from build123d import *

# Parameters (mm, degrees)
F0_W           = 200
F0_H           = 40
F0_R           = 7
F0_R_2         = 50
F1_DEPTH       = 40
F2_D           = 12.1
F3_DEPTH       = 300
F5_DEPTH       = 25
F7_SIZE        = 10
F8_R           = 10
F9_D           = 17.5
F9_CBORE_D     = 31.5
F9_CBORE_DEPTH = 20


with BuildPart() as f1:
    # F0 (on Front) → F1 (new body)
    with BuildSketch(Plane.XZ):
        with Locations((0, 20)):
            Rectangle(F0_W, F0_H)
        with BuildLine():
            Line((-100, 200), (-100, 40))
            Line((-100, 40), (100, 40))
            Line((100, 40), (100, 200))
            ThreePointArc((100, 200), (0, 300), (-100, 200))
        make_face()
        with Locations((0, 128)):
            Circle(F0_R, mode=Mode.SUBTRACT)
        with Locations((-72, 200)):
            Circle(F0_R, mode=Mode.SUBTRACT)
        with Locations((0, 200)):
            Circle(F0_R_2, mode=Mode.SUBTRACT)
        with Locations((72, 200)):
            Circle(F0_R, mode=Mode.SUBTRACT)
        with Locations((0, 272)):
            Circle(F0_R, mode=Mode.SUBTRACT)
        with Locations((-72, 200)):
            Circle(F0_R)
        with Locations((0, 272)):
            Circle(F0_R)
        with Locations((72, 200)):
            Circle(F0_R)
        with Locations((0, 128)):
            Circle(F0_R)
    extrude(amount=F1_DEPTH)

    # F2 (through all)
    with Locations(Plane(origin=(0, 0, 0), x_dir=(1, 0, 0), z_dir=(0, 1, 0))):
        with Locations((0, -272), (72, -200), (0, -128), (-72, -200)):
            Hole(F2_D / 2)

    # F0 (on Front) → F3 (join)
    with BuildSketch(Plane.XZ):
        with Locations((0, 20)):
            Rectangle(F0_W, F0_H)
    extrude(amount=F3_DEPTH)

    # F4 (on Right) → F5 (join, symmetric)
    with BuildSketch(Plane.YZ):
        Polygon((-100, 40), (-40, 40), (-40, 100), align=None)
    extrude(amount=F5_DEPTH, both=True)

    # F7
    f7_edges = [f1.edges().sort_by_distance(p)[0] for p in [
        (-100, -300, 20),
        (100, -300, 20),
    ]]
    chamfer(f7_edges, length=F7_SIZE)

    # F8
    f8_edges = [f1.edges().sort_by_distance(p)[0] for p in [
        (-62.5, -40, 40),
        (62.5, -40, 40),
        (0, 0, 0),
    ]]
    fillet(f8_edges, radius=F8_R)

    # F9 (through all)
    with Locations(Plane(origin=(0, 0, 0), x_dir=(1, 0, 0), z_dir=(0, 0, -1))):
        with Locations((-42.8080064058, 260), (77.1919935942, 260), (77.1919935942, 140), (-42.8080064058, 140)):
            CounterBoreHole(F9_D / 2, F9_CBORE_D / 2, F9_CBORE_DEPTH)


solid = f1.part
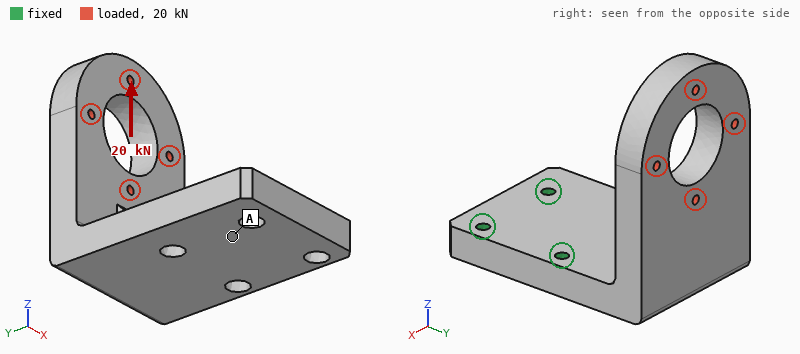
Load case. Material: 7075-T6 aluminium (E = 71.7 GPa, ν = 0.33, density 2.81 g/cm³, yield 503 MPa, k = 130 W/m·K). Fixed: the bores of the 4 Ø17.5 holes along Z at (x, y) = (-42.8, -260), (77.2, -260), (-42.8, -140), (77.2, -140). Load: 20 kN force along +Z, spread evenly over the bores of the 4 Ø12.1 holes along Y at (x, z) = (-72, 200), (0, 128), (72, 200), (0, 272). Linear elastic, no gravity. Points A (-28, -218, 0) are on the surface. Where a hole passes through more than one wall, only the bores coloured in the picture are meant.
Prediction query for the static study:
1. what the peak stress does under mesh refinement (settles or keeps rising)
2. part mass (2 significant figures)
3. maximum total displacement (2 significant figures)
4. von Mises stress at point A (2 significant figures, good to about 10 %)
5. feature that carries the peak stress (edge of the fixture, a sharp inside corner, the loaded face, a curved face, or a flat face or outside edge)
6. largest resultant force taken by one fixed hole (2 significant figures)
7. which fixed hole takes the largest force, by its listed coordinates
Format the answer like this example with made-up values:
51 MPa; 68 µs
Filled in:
keeps rising; 11 kg; 0.77 mm; 8.3 MPa; edge of the fixture; 25 kN; (-42.8, -140)
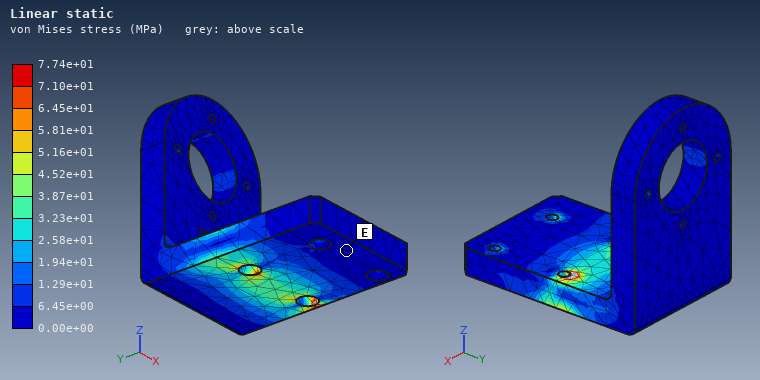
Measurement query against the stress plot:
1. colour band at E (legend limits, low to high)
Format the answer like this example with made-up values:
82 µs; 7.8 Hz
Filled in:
0.00e+00 to 6.45e+00 MPa
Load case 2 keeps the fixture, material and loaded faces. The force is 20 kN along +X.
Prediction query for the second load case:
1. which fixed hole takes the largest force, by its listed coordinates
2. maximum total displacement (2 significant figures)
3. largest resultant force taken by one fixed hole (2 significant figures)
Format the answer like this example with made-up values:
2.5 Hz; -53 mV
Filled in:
(-42.8, -140); 0.71 mm; 36 kN
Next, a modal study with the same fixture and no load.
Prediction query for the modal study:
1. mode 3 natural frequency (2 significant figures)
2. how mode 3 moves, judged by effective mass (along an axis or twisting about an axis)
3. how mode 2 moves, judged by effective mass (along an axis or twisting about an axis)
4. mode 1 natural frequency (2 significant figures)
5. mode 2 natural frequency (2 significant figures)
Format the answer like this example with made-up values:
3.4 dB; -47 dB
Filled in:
960 Hz; along Z; along X; 320 Hz; 550 Hz
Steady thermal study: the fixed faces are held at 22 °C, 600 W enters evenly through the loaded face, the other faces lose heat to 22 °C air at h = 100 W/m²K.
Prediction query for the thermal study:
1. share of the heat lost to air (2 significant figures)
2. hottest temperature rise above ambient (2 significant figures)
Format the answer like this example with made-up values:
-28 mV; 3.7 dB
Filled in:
84 %; 62 K
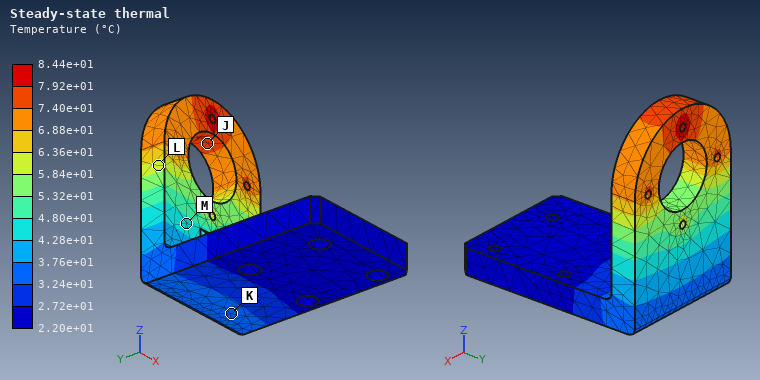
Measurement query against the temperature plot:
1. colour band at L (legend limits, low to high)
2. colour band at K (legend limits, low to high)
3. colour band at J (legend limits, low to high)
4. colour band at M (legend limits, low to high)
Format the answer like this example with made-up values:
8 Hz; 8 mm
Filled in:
5.84e+01 to 6.36e+01 °C; 3.24e+01 to 3.76e+01 °C; 7.40e+01 to 7.92e+01 °C; 4.28e+01 to 4.80e+01 °C
